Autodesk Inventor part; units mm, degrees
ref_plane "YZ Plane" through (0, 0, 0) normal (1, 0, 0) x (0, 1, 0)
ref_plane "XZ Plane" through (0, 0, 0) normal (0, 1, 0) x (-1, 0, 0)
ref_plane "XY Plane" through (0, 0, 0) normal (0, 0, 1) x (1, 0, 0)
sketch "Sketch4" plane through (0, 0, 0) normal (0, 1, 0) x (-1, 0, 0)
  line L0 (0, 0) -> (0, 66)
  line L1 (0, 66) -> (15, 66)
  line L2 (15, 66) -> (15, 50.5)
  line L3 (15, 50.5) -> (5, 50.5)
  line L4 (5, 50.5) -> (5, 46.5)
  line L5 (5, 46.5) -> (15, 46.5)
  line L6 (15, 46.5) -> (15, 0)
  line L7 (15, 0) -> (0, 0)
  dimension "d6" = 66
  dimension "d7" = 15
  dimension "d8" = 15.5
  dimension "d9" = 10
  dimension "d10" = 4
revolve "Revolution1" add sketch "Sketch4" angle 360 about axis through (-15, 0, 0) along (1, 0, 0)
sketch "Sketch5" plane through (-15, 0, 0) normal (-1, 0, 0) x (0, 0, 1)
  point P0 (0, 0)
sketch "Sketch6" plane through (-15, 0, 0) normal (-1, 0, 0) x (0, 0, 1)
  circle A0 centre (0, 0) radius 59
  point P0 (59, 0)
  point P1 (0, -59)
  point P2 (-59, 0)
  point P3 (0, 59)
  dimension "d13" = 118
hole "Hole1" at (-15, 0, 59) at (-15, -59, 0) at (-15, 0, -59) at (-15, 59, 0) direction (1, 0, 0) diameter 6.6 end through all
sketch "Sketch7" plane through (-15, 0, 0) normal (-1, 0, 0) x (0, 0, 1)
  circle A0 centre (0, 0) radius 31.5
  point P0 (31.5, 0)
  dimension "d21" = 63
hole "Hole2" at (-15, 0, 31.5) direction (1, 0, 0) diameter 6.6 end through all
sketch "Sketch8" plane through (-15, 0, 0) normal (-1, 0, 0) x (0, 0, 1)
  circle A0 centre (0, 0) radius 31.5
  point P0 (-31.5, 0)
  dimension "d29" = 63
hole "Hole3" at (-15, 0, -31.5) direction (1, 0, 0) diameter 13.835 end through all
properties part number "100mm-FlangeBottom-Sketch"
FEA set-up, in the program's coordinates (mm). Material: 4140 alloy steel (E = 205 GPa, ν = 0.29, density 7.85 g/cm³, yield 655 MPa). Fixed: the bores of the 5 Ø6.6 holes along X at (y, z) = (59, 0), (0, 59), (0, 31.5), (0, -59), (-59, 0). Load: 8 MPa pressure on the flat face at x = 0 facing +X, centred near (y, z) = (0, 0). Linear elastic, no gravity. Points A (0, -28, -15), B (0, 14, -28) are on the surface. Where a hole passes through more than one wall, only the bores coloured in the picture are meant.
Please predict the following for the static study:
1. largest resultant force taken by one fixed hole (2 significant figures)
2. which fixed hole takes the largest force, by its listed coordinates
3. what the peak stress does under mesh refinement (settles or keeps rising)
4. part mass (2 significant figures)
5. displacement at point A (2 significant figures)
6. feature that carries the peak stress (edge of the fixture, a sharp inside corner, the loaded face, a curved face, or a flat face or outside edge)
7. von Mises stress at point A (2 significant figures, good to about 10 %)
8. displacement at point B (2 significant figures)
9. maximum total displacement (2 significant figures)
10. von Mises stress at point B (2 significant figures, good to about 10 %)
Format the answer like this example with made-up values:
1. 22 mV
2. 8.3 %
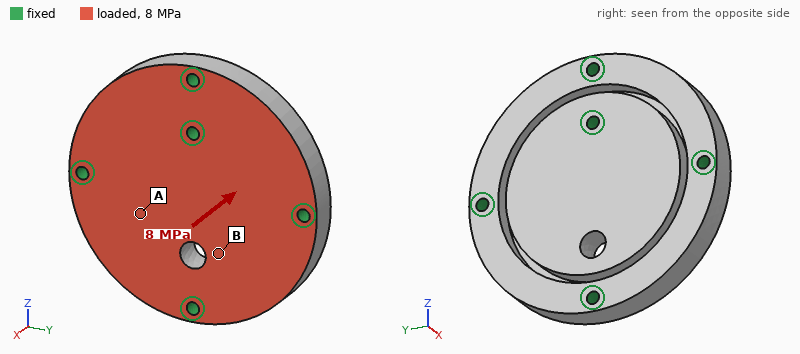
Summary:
1. 30 kN
2. (0, 31.5)
3. keeps rising
4. 1.5 kg
5. 41 µm
6. edge of the fixture
7. 35 MPa
8. 44 µm
9. 47 µm
10. 65 MPa
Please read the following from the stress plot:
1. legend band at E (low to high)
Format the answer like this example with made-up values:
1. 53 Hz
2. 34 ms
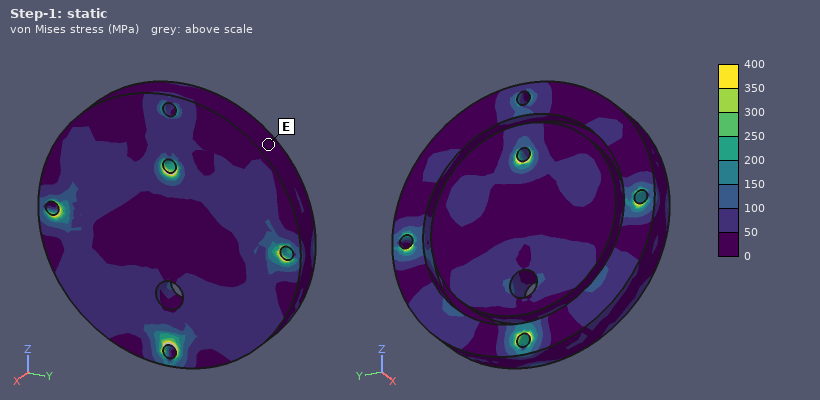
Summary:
1. 0 to 50 MPa
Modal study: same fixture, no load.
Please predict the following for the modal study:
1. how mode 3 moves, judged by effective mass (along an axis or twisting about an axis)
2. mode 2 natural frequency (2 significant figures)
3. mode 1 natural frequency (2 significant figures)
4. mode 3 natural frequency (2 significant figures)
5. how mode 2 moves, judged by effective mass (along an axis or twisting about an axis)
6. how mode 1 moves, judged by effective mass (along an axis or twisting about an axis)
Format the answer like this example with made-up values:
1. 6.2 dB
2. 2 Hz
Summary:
1. twisting about Z
2. 7800 Hz
3. 7000 Hz
4. 8400 Hz
5. twisting about Z
6. along X
